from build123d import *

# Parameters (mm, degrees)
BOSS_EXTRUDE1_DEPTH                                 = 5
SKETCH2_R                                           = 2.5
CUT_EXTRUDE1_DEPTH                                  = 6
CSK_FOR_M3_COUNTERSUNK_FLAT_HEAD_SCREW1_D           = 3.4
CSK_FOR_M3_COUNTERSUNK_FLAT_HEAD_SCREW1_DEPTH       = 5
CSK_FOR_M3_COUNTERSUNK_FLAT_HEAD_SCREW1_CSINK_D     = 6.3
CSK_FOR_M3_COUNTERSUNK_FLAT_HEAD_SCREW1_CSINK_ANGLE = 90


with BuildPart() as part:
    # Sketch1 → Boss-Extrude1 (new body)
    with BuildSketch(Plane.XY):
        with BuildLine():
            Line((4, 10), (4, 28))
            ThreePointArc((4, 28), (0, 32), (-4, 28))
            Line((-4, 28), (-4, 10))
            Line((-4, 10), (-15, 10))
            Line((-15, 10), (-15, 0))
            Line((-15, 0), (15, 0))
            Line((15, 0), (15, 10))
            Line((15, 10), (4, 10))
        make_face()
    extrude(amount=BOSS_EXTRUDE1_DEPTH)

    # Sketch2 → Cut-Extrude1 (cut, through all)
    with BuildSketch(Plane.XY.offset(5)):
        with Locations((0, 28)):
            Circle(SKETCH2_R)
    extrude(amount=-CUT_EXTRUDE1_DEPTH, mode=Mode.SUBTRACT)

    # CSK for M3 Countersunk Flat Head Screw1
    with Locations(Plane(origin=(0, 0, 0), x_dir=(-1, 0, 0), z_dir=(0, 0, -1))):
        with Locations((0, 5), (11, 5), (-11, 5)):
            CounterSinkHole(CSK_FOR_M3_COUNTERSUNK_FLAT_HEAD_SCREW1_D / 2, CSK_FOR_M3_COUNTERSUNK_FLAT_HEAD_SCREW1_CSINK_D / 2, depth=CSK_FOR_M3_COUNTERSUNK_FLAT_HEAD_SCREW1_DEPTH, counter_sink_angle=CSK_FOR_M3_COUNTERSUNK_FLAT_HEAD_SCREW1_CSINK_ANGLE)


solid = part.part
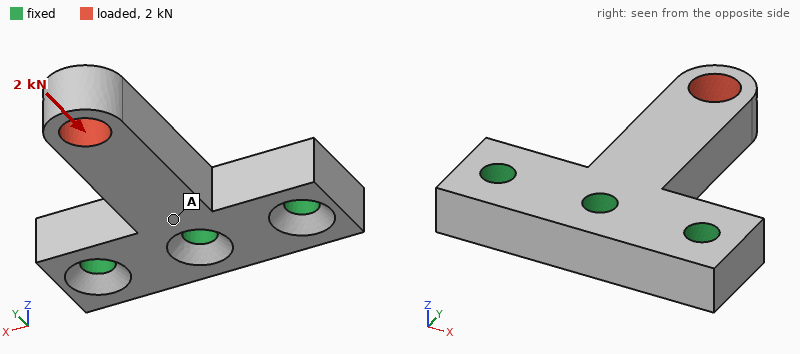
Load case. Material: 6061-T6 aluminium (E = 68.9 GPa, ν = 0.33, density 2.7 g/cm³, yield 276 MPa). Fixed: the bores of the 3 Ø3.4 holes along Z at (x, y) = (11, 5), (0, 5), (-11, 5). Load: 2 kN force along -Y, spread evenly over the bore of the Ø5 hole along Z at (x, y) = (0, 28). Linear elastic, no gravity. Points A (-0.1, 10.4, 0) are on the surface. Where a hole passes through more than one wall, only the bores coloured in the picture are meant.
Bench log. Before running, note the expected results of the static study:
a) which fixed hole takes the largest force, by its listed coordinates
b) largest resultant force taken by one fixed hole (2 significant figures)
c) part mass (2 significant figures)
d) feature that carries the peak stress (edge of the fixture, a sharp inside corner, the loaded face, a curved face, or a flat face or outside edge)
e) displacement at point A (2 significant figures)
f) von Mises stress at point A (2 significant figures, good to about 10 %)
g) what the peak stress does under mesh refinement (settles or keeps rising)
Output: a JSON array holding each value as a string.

["(0, 5)", "1.6 kN", "5.6 g", "edge of the fixture", "5.3 µm", "39 MPa", "keeps rising"]
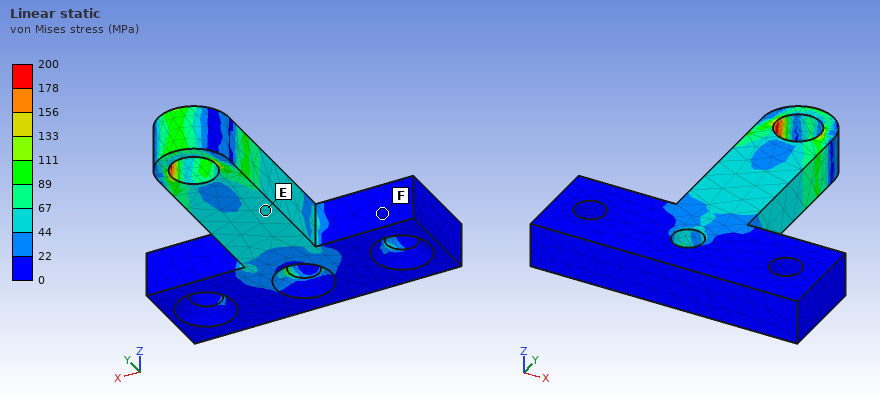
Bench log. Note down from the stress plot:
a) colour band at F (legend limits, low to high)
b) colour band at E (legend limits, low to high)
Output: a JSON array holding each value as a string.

["0 to 22 MPa", "44 to 67 MPa"]
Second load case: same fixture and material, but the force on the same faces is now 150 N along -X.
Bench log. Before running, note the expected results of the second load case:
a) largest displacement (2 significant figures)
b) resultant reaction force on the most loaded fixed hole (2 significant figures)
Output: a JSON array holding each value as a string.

["46 µm", "180 N"]
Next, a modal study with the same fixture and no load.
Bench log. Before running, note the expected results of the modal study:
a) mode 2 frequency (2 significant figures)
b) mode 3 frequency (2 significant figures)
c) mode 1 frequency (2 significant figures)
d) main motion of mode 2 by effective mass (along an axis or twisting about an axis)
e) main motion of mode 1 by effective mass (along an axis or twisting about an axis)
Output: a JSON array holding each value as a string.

["12 kHz", "29 kHz", "7100 Hz", "along X", "along Z"]
